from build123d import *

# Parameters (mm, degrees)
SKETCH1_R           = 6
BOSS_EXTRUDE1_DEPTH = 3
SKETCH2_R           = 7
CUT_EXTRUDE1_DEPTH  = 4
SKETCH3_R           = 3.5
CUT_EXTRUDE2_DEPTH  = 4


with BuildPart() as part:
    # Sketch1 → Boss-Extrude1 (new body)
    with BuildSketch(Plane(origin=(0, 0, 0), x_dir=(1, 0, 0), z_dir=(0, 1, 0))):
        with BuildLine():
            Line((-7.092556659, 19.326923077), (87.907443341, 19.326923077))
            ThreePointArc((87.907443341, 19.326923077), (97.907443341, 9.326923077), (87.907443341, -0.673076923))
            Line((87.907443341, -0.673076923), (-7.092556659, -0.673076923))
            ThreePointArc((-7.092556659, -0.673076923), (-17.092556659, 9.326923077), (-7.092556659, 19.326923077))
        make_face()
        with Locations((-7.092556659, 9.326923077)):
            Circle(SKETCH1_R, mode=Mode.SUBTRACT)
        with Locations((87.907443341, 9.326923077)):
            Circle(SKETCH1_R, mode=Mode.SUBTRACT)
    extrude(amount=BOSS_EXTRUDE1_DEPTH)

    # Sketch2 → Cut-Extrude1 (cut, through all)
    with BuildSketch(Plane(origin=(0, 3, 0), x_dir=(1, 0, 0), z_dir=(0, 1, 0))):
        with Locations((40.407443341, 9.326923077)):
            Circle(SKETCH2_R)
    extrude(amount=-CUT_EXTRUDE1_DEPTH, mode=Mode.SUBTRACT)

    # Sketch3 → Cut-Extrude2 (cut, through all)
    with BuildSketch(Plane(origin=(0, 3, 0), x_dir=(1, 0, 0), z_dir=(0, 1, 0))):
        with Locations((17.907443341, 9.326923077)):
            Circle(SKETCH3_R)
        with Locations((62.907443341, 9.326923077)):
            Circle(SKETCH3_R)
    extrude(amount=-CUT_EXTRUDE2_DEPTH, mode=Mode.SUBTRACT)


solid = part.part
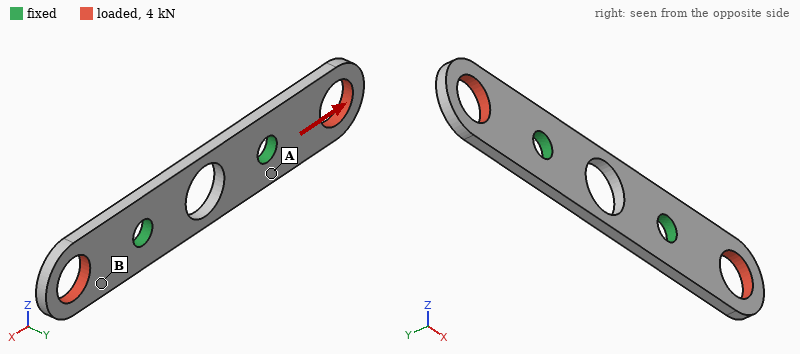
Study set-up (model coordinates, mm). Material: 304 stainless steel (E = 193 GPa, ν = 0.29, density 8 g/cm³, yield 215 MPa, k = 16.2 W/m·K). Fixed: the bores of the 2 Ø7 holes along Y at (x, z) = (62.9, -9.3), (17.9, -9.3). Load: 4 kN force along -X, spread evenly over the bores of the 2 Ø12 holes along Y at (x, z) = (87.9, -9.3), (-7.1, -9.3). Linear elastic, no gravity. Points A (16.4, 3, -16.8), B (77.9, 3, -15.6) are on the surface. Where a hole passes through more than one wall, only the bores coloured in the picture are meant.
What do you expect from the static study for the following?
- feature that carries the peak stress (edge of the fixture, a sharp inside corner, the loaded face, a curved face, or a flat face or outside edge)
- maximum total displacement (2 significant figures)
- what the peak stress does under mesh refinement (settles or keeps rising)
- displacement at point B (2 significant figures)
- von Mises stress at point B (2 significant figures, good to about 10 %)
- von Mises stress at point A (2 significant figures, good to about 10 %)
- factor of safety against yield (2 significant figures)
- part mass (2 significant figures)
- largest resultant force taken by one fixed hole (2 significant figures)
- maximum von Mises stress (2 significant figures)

the loaded face
11 µm
settles
2.9 µm
41 MPa
19 MPa
1.7
42 g
2.0 kN
130 MPa
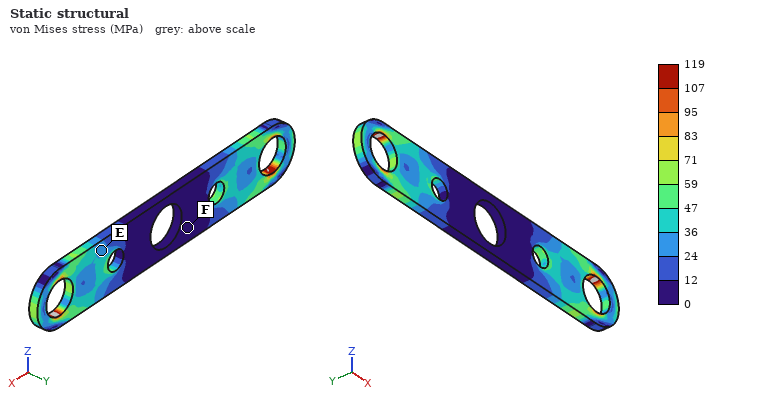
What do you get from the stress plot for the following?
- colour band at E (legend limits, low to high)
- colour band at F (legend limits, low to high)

24 to 36 MPa
0 to 12 MPa
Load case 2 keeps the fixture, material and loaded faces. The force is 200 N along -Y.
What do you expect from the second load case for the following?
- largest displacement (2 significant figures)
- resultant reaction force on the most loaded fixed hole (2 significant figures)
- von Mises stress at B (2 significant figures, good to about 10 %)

83 µm
100 N
34 MPa
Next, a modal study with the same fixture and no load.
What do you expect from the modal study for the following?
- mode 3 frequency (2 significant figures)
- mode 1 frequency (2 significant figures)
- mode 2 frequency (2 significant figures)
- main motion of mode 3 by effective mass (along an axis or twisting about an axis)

7700 Hz
2900 Hz
2900 Hz
twisting about X
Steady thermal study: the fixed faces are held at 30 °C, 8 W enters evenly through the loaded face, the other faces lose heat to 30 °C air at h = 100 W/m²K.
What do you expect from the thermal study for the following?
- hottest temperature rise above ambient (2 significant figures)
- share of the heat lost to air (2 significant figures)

52 K
72 %
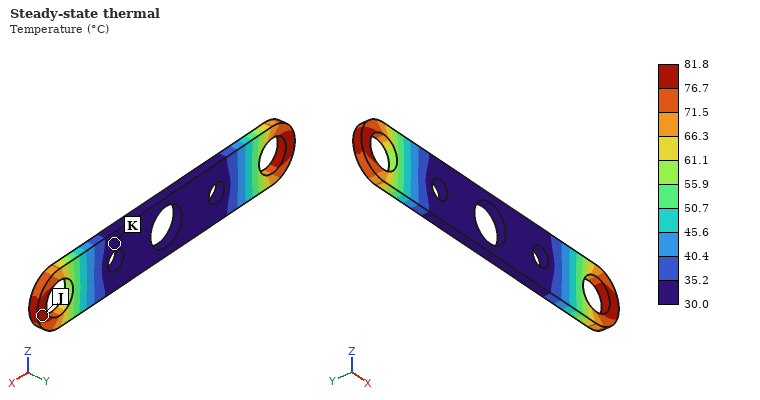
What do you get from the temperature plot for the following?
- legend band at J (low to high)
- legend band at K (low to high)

76.7 to 81.8 °C
30.0 to 35.2 °C
